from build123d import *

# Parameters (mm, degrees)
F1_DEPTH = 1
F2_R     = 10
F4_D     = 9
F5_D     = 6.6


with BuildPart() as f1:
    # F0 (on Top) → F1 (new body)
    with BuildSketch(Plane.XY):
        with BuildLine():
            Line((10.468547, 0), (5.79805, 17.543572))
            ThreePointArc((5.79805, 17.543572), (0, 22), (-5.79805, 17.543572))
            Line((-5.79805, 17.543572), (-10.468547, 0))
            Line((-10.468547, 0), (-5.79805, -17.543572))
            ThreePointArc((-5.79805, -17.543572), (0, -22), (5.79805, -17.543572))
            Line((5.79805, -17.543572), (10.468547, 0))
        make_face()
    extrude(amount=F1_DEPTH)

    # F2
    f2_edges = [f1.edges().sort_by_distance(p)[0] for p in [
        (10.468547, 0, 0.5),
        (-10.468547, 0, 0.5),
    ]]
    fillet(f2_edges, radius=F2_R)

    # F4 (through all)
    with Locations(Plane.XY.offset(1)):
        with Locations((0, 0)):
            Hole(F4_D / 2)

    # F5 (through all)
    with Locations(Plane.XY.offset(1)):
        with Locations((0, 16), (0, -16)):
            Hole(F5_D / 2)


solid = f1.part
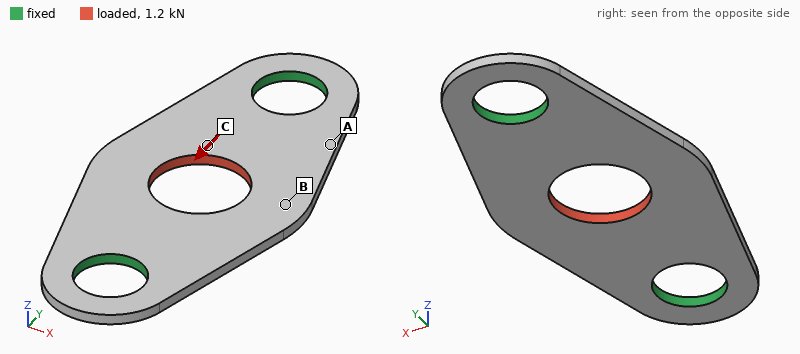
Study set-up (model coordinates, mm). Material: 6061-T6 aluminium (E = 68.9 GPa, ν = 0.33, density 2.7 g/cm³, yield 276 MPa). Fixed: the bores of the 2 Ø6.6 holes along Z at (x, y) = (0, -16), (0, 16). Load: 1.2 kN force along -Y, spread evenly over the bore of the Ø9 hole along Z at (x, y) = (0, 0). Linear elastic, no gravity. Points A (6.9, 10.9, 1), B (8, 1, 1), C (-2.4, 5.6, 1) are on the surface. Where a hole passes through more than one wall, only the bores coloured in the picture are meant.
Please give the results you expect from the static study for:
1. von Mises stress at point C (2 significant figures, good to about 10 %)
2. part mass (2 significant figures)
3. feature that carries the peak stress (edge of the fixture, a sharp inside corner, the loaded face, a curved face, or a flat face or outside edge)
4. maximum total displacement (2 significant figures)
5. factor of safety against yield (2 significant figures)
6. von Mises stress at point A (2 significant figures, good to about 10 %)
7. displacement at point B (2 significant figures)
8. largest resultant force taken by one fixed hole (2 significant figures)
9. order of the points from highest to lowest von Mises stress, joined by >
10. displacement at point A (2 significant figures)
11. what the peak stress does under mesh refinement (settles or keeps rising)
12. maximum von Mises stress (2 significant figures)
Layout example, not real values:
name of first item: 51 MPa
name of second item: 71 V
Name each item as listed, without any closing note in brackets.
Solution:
von Mises stress at point C: 57 MPa
part mass: 1.4 g
feature that carries the peak stress: the loaded face
maximum total displacement: 9.5 µm
factor of safety against yield: 3.6
von Mises stress at point A: 23 MPa
displacement at point B: 5.8 µm
largest resultant force taken by one fixed hole: 600 N
order of the points from highest to lowest von Mises stress, joined by >: C > A > B
displacement at point A: 4.3 µm
what the peak stress does under mesh refinement: settles
maximum von Mises stress: 77 MPa
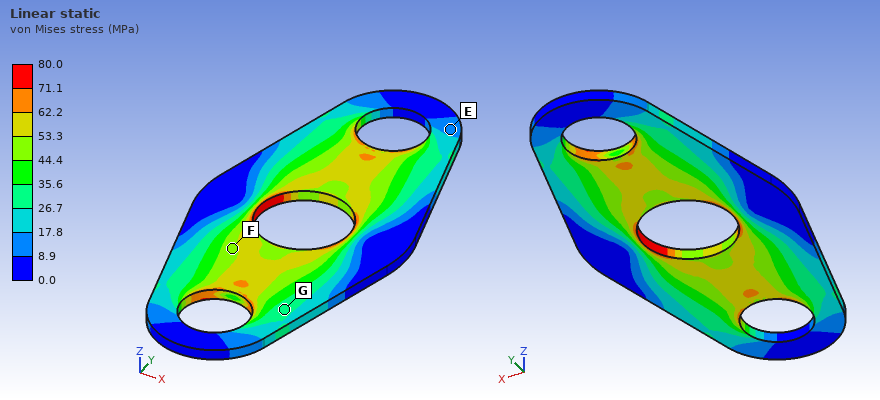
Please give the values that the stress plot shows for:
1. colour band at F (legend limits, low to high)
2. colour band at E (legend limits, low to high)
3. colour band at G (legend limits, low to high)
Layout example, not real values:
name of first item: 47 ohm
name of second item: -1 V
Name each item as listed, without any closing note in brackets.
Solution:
colour band at F: 44.4 to 53.3 MPa
colour band at E: 8.9 to 17.8 MPa
colour band at G: 26.7 to 35.6 MPa
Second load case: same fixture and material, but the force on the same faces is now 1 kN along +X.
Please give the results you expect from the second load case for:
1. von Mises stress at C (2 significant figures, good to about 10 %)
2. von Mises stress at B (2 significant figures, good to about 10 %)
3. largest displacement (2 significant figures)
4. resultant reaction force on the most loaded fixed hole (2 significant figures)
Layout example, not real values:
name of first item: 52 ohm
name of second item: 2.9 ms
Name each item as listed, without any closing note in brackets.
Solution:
von Mises stress at C: 58 MPa
von Mises stress at B: 62 MPa
largest displacement: 22 µm
resultant reaction force on the most loaded fixed hole: 500 N
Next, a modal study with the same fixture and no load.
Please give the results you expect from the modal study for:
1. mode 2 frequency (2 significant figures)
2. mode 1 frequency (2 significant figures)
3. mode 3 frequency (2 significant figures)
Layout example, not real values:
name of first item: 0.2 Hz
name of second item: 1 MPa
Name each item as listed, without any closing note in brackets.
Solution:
mode 2 frequency: 6600 Hz
mode 1 frequency: 6400 Hz
mode 3 frequency: 16 kHz
